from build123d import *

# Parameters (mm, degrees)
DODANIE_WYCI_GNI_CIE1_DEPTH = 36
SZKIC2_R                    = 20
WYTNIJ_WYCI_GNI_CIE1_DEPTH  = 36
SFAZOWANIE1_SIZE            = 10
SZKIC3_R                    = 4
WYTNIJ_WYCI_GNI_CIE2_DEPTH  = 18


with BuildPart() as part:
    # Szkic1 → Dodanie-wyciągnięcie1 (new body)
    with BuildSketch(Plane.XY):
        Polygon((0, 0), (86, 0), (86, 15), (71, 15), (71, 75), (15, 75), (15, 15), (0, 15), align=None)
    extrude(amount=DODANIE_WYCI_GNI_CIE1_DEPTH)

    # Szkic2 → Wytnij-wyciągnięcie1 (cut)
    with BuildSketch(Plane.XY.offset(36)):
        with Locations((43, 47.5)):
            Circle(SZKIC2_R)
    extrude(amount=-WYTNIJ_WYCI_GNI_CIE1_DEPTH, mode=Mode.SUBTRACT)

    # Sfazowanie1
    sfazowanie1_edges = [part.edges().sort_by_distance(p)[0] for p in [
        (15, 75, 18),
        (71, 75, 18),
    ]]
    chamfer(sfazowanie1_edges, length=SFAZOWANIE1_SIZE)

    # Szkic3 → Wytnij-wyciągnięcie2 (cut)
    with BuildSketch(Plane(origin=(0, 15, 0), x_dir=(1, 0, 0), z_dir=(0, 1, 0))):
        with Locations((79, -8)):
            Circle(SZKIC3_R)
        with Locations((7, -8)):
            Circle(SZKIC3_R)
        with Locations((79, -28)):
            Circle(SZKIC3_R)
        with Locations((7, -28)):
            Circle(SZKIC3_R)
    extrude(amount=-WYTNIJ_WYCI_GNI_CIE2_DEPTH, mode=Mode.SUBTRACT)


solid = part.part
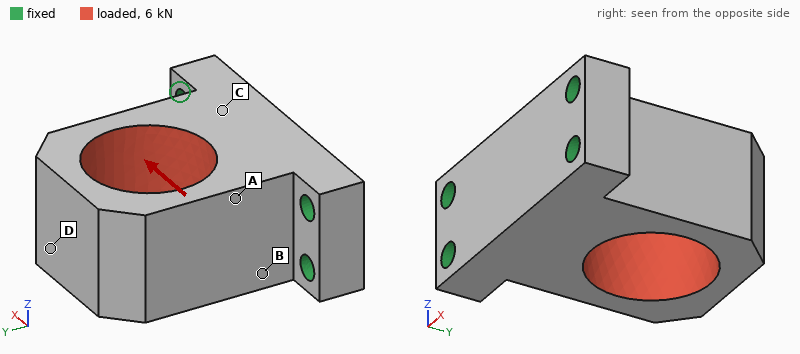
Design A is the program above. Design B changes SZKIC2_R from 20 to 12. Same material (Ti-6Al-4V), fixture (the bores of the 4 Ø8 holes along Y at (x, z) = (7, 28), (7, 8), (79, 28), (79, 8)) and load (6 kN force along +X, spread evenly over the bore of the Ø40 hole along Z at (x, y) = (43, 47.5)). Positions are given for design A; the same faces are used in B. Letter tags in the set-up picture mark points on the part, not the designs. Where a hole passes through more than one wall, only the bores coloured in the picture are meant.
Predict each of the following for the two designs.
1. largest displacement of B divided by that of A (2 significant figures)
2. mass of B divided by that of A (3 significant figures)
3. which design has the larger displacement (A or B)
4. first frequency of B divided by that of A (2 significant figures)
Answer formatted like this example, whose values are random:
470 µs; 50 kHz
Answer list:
0.40; 1.25; A; 0.90
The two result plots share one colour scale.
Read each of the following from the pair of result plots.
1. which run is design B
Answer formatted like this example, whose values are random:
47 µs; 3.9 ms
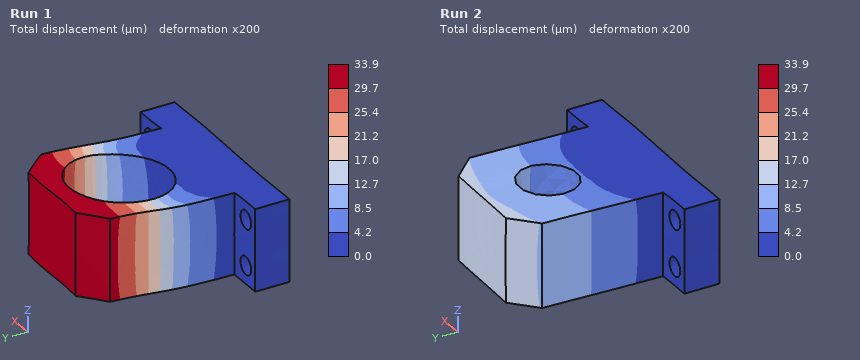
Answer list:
Run 2
